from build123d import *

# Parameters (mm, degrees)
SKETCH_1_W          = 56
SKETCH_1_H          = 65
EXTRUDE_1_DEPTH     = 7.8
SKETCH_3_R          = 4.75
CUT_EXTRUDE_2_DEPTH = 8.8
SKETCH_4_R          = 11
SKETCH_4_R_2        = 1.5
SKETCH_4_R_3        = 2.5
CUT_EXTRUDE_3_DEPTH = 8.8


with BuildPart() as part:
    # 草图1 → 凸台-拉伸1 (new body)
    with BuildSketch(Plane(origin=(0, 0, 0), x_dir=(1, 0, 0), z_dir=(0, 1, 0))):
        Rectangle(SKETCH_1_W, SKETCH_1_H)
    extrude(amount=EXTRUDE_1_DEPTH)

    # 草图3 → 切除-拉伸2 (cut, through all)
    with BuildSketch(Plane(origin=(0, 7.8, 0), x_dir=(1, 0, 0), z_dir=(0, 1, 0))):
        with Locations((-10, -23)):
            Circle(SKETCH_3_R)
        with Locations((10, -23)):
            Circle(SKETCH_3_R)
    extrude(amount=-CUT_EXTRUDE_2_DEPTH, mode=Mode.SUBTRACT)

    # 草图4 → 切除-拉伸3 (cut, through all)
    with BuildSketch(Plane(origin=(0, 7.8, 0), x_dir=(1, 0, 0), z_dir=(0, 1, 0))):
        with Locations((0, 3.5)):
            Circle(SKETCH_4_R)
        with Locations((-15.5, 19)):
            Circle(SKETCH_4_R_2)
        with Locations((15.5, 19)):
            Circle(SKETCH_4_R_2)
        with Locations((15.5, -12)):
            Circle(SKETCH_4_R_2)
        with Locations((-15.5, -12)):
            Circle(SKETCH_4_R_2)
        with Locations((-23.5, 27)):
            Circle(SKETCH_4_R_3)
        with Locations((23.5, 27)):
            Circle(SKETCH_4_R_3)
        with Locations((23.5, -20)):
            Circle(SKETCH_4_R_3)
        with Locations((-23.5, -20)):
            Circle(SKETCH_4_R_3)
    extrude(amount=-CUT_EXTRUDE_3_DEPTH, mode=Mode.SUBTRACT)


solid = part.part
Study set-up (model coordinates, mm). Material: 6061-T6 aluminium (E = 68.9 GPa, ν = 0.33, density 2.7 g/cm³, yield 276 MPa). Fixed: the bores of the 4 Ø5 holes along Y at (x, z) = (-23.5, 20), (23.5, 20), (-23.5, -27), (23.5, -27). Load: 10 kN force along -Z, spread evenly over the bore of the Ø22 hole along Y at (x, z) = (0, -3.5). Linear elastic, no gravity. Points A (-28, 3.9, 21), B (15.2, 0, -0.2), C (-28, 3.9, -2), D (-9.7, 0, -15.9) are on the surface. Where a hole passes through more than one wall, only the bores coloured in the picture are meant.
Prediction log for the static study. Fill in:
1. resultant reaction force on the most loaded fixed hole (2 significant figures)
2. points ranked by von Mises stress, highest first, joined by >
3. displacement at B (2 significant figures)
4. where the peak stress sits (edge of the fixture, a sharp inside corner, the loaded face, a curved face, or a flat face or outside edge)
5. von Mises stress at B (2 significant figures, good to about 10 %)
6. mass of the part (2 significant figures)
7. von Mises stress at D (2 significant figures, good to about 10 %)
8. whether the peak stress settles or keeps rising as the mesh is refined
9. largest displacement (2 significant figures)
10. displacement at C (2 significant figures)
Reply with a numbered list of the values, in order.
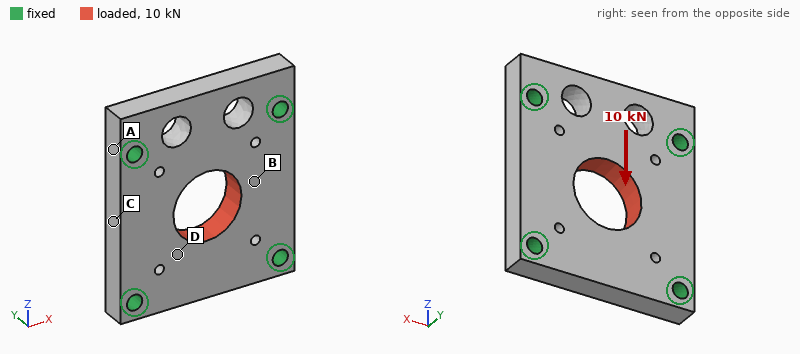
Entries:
1. 2.7 kN
2. B > D > A > C
3. 6.8 µm
4. edge of the fixture
5. 26 MPa
6. 63 g
7. 19 MPa
8. keeps rising
9. 13 µm
10. 3.4 µm
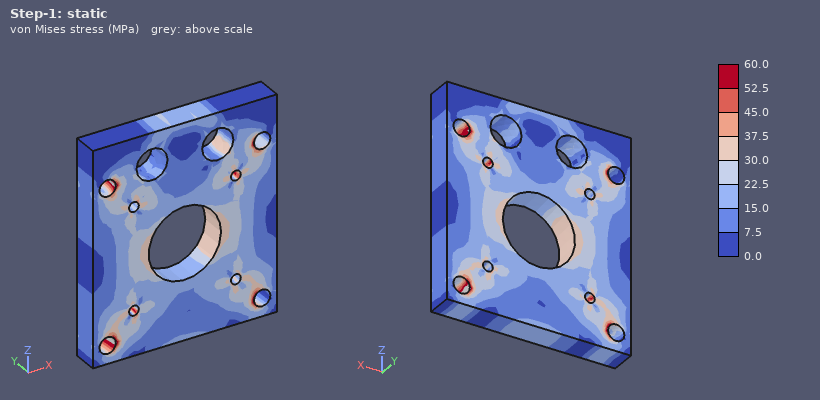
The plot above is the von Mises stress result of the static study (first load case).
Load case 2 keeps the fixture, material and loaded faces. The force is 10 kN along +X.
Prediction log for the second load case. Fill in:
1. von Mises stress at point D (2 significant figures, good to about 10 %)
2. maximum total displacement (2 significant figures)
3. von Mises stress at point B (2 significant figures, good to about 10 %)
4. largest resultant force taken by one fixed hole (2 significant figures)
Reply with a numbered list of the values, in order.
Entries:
1. 19 MPa
2. 14 µm
3. 15 MPa
4. 2.9 kN
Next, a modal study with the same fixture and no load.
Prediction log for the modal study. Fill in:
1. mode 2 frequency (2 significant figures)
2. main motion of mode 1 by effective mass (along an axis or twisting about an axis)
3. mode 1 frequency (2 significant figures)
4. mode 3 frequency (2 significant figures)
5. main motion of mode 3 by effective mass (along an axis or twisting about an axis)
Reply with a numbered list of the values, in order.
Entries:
1. 15 kHz
2. along Y
3. 12 kHz
4. 17 kHz
5. twisting about Z
